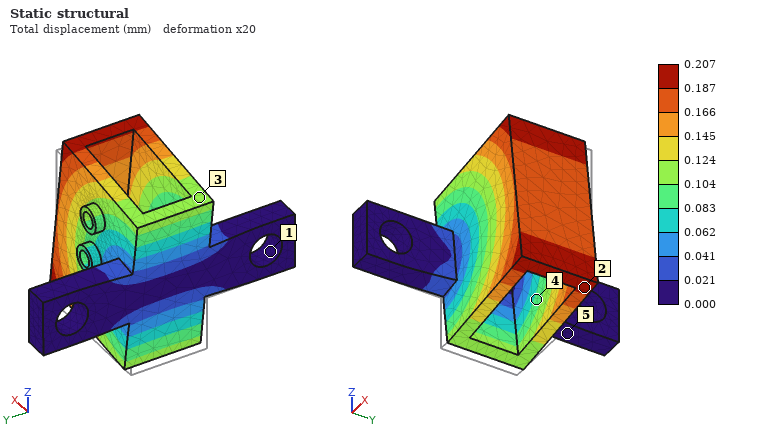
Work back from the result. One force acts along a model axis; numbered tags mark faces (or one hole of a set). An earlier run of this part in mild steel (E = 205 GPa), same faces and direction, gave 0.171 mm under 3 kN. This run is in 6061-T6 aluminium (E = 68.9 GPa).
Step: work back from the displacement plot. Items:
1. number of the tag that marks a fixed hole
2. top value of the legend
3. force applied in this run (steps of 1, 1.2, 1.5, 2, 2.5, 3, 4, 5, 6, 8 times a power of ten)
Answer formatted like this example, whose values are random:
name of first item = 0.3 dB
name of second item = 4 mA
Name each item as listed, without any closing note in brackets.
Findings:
number of the tag that marks a fixed hole = 1
top value of the legend = 0.207 mm
force applied in this run = 1.2 kN
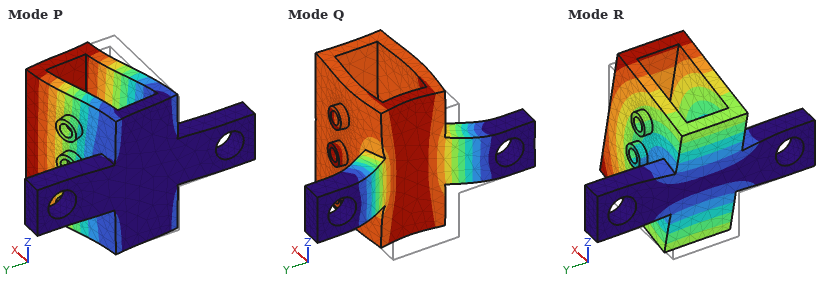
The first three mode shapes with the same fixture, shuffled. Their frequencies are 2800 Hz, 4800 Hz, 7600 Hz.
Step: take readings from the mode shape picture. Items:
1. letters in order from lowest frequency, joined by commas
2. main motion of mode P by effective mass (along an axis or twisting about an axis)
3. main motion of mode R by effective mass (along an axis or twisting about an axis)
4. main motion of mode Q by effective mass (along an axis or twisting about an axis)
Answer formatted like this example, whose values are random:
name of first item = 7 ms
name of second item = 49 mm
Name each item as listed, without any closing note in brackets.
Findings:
letters in order from lowest frequency, joined by commas = R, P, Q
main motion of mode P by effective mass = along Y
main motion of mode R by effective mass = along Z
main motion of mode Q by effective mass = along X
